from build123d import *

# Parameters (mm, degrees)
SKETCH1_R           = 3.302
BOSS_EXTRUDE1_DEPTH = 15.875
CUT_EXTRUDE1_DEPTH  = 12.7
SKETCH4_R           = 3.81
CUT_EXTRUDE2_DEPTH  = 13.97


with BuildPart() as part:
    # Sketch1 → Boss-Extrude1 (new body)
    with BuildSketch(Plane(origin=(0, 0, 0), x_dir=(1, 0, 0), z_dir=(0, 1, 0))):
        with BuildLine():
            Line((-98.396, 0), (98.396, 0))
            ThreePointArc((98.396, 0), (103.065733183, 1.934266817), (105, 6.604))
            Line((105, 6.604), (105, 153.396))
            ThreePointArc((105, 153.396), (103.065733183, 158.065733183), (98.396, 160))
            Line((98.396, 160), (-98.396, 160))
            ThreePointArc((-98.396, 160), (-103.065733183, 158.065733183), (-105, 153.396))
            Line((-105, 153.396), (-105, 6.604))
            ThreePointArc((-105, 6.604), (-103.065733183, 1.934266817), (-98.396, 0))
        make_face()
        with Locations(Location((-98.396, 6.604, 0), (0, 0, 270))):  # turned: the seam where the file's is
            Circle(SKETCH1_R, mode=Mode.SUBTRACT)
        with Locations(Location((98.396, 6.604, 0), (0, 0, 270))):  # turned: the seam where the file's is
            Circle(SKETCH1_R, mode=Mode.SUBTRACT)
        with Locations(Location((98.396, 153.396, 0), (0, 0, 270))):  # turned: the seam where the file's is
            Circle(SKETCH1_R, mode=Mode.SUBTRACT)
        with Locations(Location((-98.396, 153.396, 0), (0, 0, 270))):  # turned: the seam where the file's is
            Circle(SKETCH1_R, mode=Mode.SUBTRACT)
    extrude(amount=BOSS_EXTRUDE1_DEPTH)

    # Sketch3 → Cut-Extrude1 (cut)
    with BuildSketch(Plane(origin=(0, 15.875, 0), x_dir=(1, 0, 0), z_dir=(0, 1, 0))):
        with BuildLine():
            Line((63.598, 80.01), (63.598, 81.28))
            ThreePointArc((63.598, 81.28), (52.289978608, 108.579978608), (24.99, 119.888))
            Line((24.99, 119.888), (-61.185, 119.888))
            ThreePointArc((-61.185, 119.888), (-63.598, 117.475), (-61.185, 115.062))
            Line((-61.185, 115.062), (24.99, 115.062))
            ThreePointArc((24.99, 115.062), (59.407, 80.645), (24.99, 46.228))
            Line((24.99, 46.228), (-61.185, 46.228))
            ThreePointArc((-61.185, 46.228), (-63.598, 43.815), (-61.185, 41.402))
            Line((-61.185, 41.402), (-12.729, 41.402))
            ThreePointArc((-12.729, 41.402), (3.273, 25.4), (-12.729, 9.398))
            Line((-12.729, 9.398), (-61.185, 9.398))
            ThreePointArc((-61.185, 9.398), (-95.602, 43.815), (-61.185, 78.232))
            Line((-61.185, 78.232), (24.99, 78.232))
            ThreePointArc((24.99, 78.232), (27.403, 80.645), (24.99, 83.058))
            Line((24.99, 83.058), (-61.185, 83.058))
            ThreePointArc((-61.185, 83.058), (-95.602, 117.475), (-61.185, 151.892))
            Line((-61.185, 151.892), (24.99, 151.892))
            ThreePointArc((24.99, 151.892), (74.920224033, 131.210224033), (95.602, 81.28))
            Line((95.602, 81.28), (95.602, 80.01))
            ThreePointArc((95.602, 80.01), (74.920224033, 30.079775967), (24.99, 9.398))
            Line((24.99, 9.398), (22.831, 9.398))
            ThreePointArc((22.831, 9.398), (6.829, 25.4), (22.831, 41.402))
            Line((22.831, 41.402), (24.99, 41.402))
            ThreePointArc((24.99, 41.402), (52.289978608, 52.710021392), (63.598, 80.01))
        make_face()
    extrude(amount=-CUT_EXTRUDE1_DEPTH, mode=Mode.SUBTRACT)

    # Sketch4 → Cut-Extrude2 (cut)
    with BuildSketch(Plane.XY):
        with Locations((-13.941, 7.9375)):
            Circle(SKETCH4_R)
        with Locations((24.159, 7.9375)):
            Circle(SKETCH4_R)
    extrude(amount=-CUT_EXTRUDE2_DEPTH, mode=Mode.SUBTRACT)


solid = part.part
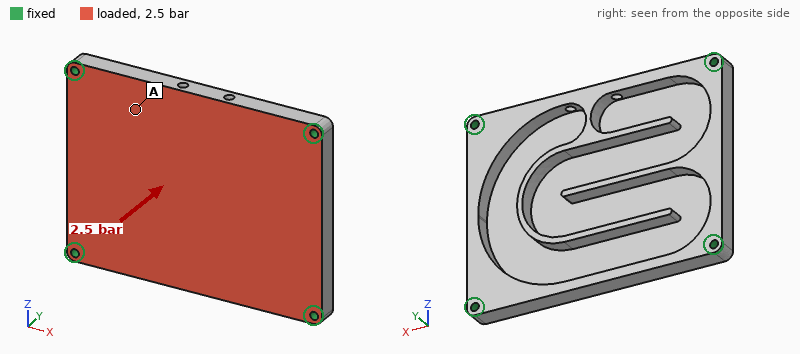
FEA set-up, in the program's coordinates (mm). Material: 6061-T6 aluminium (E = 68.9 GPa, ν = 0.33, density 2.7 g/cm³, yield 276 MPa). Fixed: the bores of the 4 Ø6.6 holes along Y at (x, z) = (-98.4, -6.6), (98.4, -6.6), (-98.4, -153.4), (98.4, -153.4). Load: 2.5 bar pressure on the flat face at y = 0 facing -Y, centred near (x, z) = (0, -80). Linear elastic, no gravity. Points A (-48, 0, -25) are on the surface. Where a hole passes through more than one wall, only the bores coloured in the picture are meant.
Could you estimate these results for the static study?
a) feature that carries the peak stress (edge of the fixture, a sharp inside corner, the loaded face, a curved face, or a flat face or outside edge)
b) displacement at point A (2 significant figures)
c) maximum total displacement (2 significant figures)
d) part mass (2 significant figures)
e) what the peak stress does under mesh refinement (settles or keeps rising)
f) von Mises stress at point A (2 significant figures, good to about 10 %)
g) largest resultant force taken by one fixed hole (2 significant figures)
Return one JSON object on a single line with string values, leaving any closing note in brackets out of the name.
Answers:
{"feature that carries the peak stress": "edge of the fixture", "displacement at point A": "0.18 mm", "maximum total displacement": "0.51 mm", "part mass": "680 g", "what the peak stress does under mesh refinement": "keeps rising", "von Mises stress at point A": "15 MPa", "largest resultant force taken by one fixed hole": "2.7 kN"}
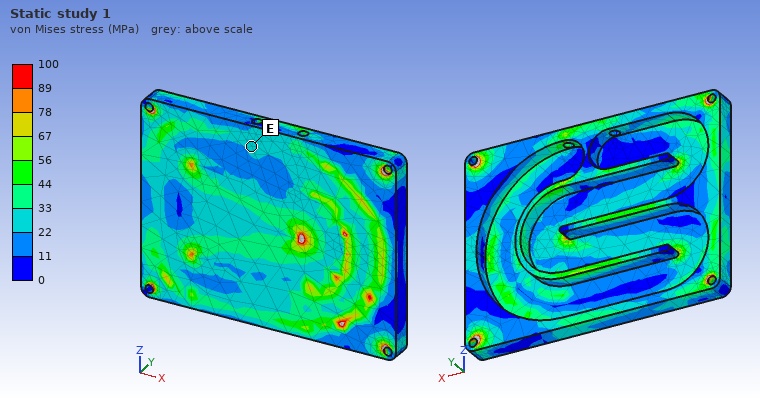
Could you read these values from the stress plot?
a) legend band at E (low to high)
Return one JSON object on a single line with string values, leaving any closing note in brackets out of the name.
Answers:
{"legend band at E": "22 to 33 MPa"}
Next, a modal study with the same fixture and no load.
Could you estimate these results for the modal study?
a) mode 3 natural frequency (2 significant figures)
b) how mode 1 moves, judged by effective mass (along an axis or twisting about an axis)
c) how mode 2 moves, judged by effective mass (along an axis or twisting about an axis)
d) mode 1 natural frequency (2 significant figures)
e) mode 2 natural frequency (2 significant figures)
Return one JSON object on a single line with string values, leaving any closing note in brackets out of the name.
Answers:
{"mode 3 natural frequency": "2300 Hz", "how mode 1 moves, judged by effective mass": "along Y", "how mode 2 moves, judged by effective mass": "twisting about X", "mode 1 natural frequency": "1200 Hz", "mode 2 natural frequency": "1800 Hz"}
